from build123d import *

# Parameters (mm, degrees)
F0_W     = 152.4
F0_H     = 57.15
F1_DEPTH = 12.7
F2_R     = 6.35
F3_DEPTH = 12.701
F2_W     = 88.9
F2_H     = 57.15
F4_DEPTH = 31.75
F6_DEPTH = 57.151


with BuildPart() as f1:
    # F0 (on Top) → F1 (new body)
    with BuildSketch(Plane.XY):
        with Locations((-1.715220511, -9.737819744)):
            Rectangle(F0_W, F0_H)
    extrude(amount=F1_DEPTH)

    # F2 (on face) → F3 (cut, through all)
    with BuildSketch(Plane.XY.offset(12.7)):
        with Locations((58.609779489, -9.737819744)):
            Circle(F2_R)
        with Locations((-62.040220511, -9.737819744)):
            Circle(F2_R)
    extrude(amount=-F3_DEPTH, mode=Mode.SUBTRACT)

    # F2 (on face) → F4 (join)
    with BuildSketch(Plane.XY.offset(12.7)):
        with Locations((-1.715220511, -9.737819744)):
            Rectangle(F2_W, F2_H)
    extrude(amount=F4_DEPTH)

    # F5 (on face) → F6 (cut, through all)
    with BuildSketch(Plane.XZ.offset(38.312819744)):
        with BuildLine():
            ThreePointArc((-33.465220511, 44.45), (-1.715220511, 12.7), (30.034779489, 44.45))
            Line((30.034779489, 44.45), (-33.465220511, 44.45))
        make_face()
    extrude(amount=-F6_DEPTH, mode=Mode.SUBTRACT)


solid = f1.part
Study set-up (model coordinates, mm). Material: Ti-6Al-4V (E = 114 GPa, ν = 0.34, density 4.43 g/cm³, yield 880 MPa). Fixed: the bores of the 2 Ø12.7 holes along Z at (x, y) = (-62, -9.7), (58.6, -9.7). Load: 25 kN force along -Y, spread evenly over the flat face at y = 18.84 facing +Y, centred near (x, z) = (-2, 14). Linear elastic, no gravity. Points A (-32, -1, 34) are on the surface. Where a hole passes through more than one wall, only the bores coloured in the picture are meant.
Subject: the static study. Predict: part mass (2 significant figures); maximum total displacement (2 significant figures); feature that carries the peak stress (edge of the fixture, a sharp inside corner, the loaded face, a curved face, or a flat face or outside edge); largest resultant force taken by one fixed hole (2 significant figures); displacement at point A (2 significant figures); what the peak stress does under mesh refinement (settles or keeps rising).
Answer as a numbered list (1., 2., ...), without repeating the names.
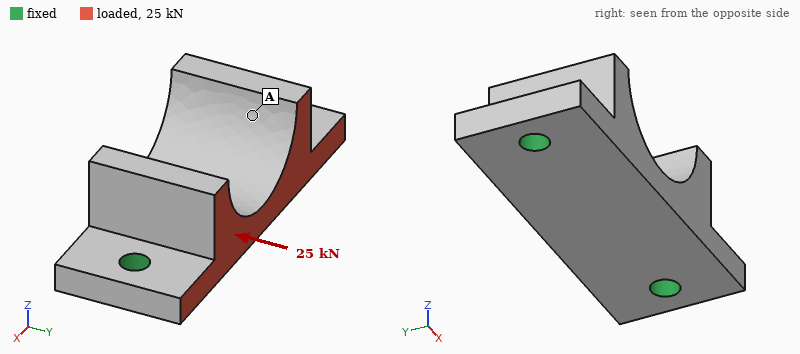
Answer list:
1. 790 g
2. 61 µm
3. edge of the fixture
4. 13 kN
5. 43 µm
6. keeps rising
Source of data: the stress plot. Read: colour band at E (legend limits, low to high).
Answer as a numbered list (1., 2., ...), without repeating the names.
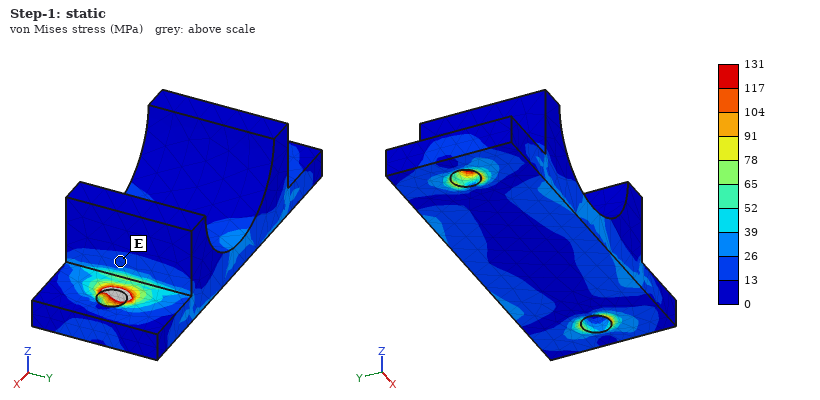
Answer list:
1. 13 to 26 MPa
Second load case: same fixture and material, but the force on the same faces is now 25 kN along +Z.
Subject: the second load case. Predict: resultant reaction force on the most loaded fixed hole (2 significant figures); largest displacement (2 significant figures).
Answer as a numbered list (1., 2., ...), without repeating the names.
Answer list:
1. 13 kN
2. 0.20 mm
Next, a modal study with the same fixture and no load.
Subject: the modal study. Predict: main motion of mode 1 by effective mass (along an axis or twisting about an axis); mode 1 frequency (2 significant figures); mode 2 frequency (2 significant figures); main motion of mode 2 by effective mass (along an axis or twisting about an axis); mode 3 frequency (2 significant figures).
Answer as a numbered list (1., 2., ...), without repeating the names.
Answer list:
1. along Z
2. 3400 Hz
3. 3700 Hz
4. along Y
5. 6300 Hz
